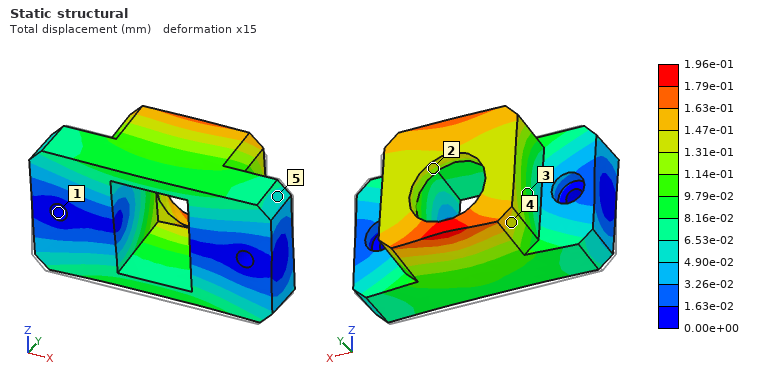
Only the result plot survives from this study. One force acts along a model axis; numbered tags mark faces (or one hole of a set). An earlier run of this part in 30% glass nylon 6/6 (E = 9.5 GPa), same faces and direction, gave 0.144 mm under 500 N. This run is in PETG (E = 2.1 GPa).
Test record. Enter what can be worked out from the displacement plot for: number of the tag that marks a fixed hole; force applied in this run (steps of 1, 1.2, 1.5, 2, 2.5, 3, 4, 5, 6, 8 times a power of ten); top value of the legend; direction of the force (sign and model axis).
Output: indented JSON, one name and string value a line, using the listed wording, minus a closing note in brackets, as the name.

{
  "number of the tag that marks a fixed hole": "1",
  "force applied in this run": "150 N",
  "top value of the legend": "1.96e-01 mm",
  "direction of the force": "+Z"
}
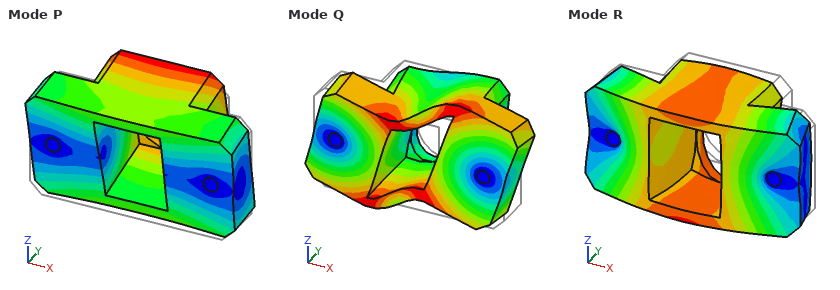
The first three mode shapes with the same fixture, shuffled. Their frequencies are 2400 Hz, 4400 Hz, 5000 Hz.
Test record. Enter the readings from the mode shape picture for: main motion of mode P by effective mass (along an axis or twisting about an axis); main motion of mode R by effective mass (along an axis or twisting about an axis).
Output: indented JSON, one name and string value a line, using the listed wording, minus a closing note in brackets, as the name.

{
  "main motion of mode P by effective mass": "along Z",
  "main motion of mode R by effective mass": "along Y"
}
